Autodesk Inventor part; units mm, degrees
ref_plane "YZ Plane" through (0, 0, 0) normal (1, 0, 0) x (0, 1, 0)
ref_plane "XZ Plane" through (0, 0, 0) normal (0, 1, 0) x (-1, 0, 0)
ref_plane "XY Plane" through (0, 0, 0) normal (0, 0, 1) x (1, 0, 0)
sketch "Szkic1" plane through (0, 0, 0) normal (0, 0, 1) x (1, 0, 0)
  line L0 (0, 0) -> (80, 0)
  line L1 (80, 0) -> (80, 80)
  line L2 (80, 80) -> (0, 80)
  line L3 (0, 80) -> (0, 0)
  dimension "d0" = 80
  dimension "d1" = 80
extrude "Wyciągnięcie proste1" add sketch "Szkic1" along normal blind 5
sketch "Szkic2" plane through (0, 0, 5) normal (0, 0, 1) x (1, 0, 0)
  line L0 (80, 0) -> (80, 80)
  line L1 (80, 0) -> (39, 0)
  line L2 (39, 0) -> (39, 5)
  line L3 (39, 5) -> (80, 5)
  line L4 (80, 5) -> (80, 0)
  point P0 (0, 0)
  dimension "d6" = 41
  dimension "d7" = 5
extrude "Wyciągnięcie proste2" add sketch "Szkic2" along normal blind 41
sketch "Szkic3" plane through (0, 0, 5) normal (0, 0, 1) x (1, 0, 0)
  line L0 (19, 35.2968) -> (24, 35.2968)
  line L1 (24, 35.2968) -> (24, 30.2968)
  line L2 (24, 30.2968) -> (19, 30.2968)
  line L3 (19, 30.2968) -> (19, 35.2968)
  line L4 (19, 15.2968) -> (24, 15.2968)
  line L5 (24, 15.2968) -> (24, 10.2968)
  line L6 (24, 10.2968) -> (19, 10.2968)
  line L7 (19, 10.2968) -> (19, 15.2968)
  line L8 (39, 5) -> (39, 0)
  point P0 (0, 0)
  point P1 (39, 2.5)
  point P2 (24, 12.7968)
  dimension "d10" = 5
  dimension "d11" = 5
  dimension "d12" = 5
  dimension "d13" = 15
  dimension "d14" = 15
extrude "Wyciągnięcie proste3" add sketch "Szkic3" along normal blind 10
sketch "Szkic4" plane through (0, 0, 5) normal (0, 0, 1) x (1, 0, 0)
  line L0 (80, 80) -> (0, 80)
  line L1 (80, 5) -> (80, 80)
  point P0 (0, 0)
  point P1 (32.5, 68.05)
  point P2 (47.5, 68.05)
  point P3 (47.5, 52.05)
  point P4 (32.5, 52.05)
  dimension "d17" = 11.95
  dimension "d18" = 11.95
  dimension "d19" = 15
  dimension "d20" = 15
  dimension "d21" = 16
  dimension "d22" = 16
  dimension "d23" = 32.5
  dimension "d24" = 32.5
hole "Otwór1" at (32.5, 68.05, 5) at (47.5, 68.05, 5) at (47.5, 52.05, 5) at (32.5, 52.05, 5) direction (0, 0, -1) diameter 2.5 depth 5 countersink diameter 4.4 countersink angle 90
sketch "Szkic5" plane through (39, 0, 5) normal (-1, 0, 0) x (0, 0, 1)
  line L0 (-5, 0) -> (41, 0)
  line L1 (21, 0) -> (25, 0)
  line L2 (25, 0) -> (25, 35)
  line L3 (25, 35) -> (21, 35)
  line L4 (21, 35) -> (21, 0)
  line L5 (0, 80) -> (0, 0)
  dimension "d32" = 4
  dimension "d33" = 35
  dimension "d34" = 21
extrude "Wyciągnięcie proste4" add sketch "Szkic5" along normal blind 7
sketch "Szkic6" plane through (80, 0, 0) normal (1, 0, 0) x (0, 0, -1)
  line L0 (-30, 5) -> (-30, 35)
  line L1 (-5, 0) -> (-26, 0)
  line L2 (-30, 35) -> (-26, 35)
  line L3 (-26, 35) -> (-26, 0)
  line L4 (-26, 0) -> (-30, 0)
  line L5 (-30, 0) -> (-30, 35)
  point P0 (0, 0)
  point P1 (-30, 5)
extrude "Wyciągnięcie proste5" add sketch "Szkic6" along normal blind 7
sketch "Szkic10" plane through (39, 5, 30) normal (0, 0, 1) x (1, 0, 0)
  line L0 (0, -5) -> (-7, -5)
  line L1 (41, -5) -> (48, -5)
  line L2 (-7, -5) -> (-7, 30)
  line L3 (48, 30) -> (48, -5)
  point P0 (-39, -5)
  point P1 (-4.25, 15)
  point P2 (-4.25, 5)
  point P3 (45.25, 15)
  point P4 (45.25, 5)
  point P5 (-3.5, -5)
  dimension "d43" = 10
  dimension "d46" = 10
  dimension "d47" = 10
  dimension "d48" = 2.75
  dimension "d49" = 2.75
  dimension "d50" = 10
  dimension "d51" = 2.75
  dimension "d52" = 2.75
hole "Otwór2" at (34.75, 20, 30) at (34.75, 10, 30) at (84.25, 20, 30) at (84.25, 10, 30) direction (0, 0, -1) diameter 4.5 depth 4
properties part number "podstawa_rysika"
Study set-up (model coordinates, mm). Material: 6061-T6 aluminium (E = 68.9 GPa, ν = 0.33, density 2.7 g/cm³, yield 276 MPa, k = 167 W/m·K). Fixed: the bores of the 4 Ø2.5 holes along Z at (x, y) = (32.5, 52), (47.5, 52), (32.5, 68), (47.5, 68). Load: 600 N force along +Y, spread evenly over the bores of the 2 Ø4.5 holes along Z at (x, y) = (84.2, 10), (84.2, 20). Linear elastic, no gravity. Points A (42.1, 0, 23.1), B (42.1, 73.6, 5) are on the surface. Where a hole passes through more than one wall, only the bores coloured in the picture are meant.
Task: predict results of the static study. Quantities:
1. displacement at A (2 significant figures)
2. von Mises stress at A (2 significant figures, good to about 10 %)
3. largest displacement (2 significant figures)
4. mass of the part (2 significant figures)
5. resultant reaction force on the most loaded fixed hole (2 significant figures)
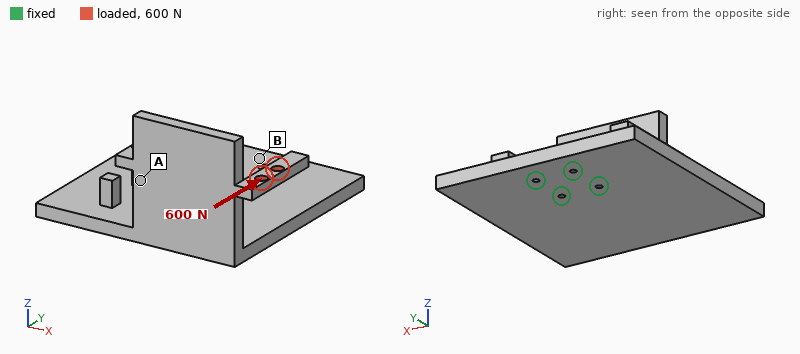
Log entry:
0.55 mm
43 MPa
1.3 mm
110 g
810 N
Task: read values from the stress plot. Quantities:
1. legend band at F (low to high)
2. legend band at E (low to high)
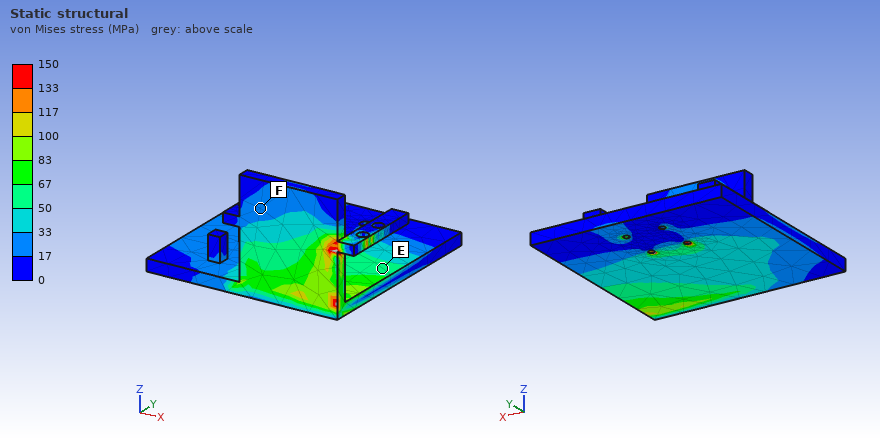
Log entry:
17 to 33 MPa
50 to 67 MPa
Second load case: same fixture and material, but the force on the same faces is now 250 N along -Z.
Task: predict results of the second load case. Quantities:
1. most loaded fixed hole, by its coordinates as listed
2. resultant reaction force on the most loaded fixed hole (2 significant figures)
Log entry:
(47.5, 52)
830 N
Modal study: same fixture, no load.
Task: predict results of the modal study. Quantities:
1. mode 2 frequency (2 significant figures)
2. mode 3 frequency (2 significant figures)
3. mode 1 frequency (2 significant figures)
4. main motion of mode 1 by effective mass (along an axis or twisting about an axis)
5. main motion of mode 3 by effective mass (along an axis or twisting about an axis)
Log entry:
1000 Hz
1400 Hz
650 Hz
along Z
along Z
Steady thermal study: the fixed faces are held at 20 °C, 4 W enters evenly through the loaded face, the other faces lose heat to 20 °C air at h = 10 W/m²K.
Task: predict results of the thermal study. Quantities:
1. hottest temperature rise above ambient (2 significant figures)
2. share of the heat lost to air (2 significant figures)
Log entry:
28 K
16 %
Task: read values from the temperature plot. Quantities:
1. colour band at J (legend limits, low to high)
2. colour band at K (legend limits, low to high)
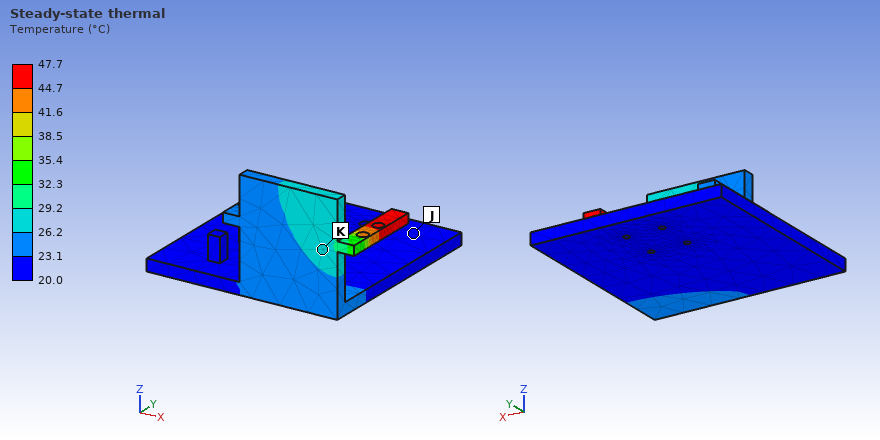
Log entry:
20.0 to 23.1 °C
26.2 to 29.2 °C
